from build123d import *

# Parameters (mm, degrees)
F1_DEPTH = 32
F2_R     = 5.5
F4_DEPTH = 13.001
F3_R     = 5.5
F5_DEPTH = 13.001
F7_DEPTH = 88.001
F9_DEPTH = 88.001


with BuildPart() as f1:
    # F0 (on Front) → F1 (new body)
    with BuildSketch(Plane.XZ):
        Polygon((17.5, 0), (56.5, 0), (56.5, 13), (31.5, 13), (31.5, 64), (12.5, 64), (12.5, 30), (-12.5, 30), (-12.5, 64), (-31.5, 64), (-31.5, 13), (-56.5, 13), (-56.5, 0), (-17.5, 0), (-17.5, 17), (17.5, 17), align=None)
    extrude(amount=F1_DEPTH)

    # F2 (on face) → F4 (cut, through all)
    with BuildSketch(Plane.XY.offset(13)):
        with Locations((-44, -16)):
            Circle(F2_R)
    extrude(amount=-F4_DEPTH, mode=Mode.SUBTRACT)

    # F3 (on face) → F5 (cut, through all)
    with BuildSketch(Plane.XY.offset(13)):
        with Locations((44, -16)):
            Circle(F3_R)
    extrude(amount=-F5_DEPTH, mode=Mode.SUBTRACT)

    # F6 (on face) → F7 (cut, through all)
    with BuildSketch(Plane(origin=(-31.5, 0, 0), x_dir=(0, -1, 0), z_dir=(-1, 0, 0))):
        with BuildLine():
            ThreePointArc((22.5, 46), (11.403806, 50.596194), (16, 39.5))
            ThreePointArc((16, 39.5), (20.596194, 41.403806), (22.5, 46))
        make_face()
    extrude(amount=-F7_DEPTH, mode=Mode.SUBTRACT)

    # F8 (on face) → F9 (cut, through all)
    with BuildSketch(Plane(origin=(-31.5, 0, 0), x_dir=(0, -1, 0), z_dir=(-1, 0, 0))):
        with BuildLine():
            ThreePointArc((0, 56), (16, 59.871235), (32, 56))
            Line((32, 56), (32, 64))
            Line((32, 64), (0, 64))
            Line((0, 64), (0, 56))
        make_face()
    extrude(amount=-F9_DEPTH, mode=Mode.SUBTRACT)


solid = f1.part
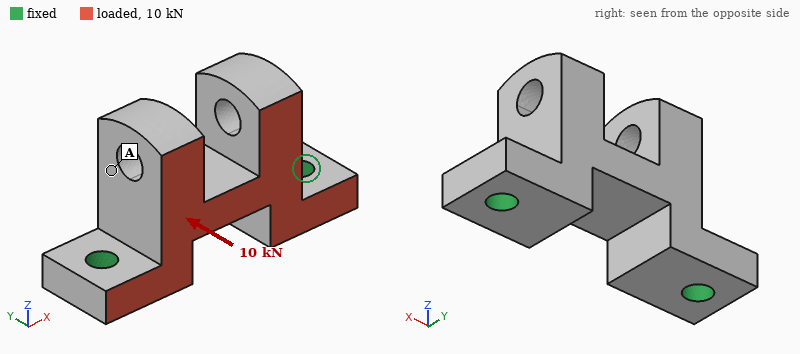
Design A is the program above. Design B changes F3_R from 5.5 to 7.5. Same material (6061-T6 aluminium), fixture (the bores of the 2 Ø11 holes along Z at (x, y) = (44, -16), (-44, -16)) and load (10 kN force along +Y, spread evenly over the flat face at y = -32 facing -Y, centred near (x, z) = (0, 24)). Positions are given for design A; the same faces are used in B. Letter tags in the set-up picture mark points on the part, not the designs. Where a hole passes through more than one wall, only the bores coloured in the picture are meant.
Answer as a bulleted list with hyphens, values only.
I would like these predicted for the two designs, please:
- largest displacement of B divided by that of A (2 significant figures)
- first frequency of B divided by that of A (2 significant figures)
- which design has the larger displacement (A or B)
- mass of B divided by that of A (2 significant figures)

- 0.90
- 1.1
- A
- 0.99
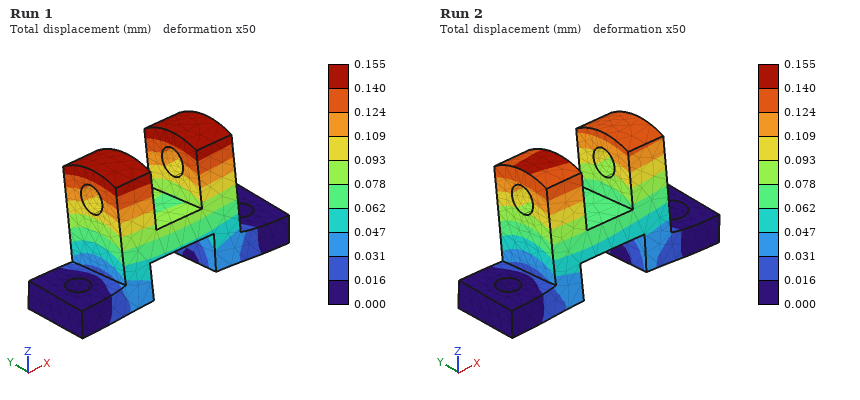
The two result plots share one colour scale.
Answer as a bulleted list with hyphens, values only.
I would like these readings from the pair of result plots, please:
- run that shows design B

- Run 2
